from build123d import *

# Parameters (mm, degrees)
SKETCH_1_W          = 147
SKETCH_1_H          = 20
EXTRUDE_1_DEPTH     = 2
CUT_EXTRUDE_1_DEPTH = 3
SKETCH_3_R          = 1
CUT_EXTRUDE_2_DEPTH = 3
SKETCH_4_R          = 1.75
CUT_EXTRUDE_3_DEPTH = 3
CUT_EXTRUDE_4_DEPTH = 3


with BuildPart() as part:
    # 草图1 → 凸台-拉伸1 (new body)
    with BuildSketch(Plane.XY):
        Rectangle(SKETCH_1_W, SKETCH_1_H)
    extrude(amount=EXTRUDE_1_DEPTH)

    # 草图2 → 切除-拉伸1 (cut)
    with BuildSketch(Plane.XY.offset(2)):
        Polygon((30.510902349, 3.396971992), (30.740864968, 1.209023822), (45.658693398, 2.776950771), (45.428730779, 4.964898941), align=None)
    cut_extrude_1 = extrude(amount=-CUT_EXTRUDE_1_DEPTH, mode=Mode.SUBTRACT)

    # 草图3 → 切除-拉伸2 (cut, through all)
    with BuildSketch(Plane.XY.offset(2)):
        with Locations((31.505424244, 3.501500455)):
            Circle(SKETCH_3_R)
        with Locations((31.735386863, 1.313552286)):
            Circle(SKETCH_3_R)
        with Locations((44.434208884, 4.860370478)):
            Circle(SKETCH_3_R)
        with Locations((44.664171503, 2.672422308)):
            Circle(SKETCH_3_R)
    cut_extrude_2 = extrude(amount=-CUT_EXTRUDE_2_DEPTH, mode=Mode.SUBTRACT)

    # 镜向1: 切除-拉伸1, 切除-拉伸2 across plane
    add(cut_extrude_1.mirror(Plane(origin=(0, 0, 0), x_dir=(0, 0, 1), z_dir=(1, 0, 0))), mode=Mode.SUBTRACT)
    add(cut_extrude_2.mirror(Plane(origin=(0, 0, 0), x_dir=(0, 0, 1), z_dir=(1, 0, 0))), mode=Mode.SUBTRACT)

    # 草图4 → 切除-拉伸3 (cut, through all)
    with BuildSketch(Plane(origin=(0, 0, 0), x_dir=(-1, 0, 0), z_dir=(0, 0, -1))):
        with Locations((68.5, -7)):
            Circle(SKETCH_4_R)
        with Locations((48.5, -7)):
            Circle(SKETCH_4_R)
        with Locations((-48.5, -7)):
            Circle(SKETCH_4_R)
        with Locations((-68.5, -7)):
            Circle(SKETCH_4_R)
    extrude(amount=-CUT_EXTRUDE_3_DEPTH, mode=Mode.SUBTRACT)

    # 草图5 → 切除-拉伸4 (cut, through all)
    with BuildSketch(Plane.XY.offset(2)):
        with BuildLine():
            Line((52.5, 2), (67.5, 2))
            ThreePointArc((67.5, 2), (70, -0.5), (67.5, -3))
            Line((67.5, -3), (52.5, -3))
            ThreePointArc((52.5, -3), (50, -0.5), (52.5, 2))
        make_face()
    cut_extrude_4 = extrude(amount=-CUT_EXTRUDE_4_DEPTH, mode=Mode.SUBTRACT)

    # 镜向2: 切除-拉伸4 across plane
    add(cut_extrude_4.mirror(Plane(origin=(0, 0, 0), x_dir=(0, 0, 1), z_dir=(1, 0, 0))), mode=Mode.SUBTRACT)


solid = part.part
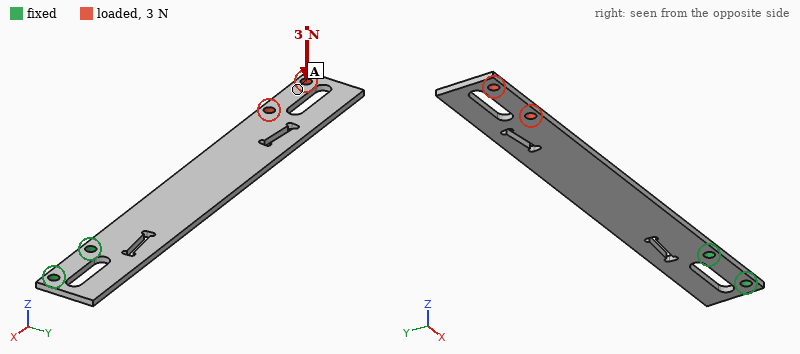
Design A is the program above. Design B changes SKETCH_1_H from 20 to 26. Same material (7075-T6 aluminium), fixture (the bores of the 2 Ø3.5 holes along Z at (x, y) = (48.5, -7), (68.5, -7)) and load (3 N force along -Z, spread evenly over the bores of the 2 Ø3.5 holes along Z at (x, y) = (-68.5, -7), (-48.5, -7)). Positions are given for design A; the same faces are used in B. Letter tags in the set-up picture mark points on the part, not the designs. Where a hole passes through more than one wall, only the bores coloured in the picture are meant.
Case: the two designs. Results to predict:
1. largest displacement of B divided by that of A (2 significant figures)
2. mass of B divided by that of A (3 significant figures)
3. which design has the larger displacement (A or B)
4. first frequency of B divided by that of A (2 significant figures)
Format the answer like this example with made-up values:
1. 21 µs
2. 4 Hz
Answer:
1. 0.76
2. 1.33
3. A
4. 0.99
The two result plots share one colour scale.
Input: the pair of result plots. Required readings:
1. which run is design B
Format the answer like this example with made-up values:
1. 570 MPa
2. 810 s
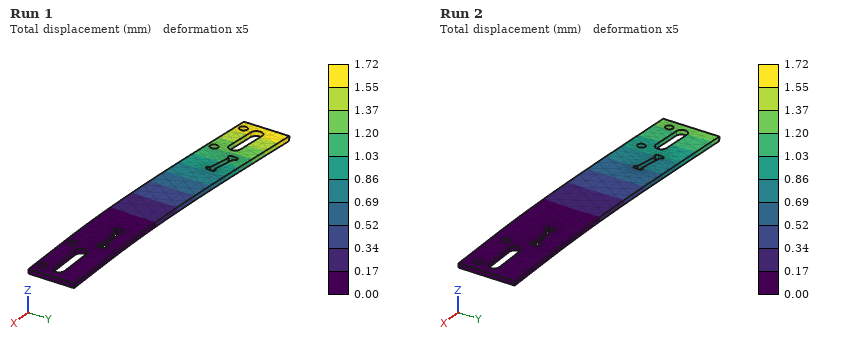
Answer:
1. Run 2
